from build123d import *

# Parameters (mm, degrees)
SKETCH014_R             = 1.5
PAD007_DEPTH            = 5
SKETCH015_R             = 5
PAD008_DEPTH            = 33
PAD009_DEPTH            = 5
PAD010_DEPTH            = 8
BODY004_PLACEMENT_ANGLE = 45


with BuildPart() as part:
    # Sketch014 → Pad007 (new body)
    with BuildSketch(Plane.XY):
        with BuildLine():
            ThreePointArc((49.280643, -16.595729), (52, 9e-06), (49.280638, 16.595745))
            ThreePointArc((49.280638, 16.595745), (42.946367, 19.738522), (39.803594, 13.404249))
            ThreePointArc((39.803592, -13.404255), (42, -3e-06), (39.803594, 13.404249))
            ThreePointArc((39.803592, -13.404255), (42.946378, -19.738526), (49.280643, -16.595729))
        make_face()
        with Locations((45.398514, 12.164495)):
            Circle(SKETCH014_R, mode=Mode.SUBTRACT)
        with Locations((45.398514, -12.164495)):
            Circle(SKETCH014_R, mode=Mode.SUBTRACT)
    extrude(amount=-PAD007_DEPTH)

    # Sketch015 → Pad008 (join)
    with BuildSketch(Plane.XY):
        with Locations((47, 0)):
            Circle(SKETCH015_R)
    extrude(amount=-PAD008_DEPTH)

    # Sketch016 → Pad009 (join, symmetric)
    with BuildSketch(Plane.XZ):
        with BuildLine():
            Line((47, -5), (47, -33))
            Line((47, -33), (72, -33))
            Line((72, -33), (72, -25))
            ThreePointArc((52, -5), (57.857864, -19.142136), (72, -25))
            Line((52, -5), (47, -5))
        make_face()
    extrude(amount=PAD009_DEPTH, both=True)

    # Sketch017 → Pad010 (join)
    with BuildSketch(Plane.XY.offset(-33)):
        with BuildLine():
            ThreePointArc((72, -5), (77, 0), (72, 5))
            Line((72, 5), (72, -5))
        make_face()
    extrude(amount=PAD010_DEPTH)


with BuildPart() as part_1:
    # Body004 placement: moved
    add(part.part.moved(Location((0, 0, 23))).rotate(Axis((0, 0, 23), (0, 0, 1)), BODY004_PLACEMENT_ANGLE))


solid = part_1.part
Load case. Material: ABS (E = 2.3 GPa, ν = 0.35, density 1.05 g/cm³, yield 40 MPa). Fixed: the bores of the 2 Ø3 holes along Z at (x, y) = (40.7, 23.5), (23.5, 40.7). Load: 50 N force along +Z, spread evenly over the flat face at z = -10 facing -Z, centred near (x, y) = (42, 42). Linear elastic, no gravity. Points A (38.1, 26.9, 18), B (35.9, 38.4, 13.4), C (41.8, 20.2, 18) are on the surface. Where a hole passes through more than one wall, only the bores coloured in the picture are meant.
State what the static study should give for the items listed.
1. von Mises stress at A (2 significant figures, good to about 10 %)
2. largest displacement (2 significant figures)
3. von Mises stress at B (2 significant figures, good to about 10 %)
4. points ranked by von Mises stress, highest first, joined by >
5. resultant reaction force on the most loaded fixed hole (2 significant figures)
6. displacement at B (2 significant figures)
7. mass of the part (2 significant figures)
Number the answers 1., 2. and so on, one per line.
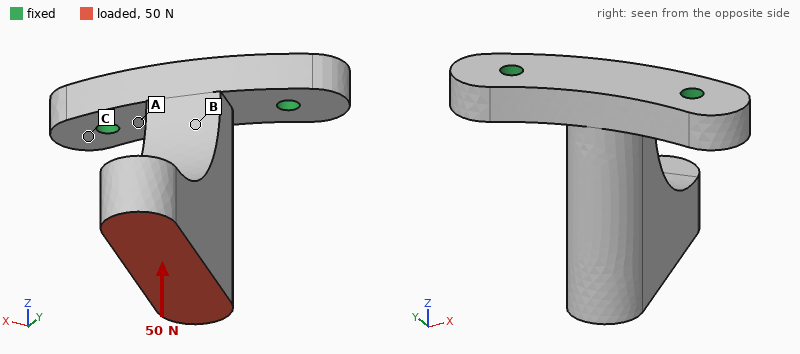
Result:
1. 7.0 MPa
2. 0.67 mm
3. 4.6 MPa
4. A > B > C
5. 25 N
6. 0.13 mm
7. 7.5 g
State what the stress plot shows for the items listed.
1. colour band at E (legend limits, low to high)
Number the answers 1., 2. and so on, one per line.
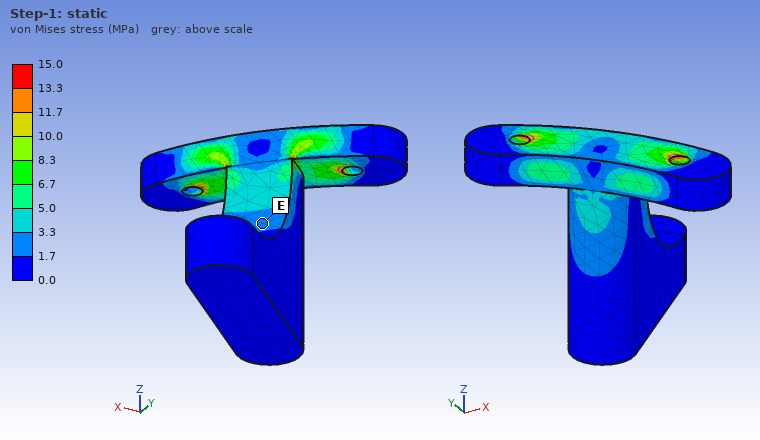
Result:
1. 1.7 to 3.3 MPa
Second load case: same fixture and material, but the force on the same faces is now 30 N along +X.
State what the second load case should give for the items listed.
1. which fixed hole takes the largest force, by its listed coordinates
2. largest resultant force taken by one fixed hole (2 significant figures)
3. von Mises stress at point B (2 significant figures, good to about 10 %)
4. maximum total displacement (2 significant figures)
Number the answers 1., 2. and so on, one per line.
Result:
1. (23.5, 40.7)
2. 47 N
3. 2.5 MPa
4. 0.67 mm
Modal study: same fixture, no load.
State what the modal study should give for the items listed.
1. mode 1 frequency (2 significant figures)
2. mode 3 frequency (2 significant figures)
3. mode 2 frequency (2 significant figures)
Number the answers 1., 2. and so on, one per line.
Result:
1. 590 Hz
2. 2300 Hz
3. 970 Hz
